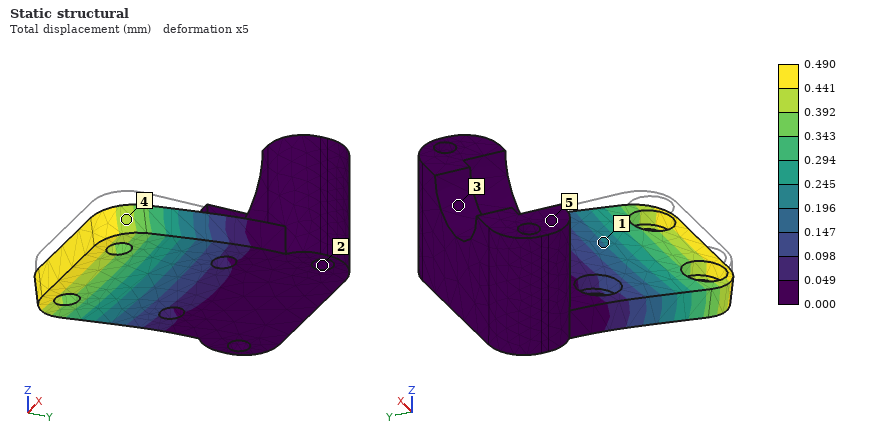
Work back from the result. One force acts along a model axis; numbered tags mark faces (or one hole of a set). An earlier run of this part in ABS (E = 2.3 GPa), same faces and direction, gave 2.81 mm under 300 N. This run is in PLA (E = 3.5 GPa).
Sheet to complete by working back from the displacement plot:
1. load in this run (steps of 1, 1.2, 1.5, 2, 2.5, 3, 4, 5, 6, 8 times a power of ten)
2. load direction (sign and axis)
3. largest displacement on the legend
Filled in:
80 N
-Z
0.490 mm
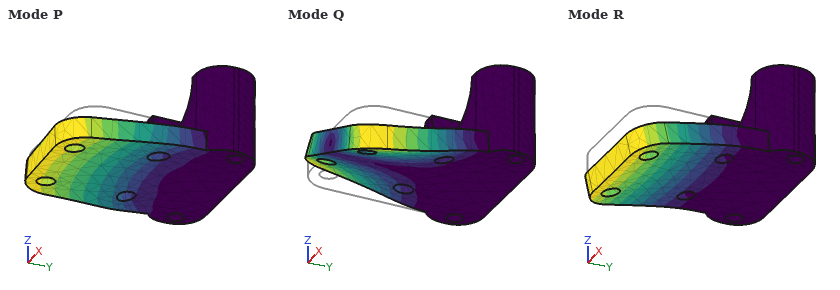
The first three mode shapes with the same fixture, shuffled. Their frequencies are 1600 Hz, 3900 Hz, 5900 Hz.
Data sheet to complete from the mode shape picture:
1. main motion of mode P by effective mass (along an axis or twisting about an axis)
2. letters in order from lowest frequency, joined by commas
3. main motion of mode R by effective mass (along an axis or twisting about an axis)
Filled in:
along X
R, Q, P
along Z
